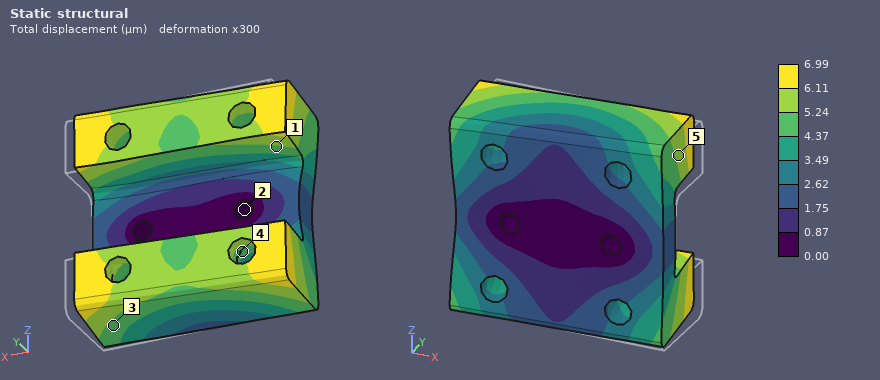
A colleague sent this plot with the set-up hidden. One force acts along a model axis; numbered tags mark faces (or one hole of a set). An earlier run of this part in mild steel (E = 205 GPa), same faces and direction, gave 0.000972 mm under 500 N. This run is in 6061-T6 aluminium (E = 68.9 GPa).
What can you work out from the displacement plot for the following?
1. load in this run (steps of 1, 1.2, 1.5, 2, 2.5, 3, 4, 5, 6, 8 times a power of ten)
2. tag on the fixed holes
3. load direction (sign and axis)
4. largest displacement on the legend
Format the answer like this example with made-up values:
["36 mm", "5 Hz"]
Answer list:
["1.2 kN", "2", "-X", "6.99 µm"]
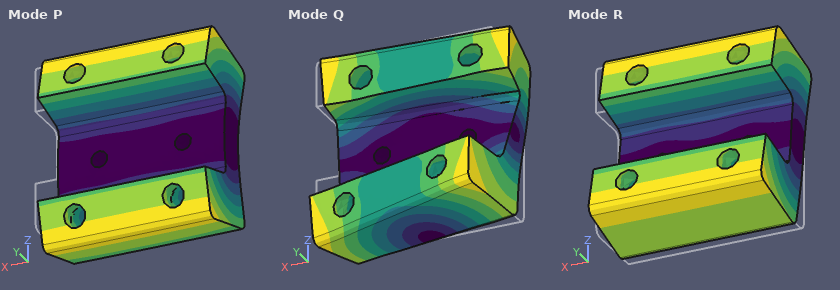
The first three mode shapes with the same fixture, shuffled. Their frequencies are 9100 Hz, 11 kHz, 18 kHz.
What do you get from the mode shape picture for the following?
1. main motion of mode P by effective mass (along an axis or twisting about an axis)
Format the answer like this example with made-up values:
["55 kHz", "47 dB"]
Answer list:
["along Y"]
